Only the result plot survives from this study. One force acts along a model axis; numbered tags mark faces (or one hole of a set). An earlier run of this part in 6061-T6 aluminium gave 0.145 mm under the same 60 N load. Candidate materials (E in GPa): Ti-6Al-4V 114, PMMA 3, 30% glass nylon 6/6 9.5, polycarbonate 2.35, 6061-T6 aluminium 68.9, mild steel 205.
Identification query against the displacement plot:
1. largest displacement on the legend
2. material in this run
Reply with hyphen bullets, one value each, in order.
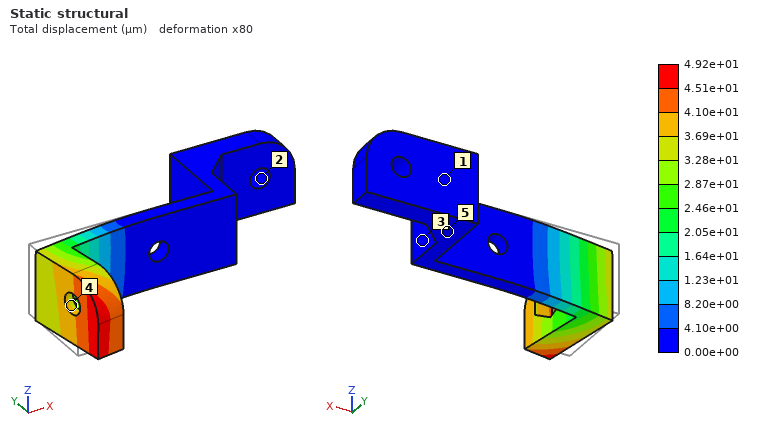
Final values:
- 4.92e+01 µm
- mild steel
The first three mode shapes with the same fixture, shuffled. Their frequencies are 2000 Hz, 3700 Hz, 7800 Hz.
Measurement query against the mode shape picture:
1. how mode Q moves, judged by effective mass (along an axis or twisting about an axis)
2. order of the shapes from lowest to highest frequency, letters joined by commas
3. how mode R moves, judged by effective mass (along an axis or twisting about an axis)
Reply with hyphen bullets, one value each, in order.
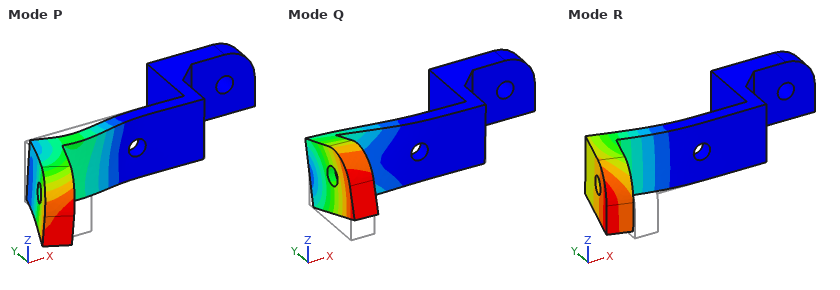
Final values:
- along Z
- R, Q, P
- along Y
